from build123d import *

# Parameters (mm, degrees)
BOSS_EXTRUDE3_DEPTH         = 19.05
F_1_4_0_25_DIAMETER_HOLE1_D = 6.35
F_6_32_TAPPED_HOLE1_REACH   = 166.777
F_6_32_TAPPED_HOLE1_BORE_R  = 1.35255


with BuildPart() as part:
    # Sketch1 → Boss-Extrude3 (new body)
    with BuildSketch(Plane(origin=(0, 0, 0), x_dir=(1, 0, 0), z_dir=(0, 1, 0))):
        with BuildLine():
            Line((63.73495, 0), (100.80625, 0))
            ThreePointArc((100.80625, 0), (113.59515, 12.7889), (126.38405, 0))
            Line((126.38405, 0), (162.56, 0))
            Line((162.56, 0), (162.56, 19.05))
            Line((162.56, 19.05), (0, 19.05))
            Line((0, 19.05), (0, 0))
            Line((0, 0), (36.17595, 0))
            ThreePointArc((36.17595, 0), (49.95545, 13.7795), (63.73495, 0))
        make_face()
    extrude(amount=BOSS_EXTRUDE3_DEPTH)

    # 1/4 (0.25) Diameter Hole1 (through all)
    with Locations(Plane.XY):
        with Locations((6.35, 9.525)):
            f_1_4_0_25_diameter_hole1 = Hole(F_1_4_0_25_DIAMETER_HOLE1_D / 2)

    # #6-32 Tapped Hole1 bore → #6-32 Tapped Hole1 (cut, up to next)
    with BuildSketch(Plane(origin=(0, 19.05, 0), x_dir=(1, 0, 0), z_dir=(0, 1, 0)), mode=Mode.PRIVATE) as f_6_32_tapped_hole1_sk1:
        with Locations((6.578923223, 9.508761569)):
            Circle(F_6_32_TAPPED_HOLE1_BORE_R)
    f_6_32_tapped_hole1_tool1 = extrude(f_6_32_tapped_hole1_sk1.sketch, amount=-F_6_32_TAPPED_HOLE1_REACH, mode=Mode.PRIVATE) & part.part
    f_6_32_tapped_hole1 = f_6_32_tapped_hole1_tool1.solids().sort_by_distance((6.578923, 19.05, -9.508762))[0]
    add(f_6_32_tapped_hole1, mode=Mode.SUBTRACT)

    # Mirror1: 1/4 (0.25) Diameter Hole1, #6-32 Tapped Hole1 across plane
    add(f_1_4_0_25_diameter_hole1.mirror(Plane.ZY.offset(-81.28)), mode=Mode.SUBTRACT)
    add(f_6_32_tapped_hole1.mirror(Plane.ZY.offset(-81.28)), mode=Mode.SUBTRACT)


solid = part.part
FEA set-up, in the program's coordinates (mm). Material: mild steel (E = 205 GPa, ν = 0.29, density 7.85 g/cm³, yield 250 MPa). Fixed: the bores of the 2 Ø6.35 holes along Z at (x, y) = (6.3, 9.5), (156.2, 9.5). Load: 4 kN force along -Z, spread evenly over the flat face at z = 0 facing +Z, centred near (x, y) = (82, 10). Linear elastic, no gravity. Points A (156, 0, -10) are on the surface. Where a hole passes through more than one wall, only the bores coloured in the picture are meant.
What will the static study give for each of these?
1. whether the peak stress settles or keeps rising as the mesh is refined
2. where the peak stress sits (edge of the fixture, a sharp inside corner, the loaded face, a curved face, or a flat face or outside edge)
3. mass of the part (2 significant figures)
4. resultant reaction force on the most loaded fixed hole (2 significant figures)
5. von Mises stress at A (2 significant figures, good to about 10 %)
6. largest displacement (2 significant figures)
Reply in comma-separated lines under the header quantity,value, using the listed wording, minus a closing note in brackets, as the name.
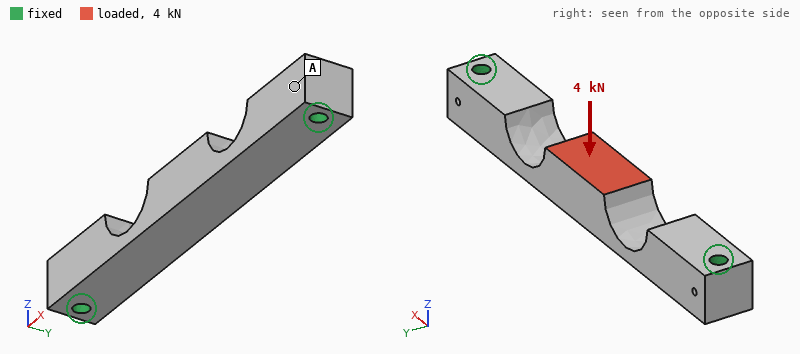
quantity,value
whether the peak stress settles or keeps rising as the mesh is refined,keeps rising
where the peak stress sits,edge of the fixture
mass of the part,370 g
resultant reaction force on the most loaded fixed hole,2.3 kN
von Mises stress at A,16 MPa
largest displacement,55 µm
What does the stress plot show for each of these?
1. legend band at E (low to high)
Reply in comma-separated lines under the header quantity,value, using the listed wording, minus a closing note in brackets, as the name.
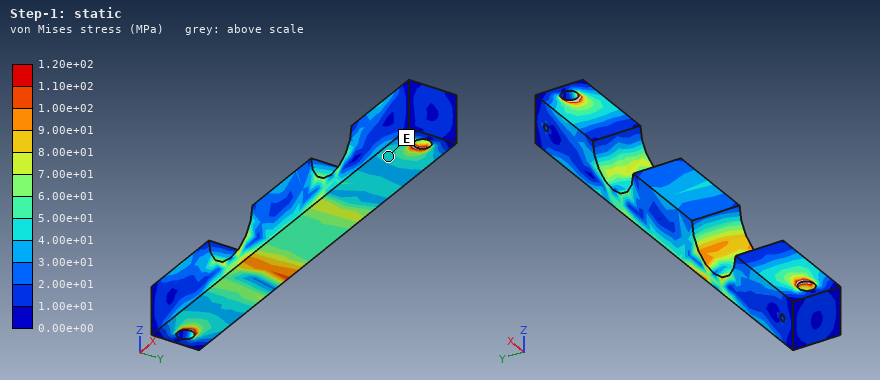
quantity,value
legend band at E,4.00e+01 to 5.00e+01 MPa
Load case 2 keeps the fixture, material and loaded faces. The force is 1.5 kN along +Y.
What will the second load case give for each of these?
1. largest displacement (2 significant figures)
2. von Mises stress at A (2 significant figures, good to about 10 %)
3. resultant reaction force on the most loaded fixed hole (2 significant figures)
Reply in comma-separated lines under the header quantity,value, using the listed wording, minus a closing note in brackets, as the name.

quantity,value
largest displacement,55 µm
von Mises stress at A,12 MPa
resultant reaction force on the most loaded fixed hole,770 N
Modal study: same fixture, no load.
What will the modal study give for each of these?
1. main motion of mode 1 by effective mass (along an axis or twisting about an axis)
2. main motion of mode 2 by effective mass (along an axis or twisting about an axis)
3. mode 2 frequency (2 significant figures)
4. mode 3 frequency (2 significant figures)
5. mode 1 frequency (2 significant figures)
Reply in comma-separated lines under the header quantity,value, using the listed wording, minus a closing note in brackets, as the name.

quantity,value
main motion of mode 1 by effective mass,along Y
main motion of mode 2 by effective mass,along Z
mode 2 frequency,3700 Hz
mode 3 frequency,6400 Hz
mode 1 frequency,3300 Hz
